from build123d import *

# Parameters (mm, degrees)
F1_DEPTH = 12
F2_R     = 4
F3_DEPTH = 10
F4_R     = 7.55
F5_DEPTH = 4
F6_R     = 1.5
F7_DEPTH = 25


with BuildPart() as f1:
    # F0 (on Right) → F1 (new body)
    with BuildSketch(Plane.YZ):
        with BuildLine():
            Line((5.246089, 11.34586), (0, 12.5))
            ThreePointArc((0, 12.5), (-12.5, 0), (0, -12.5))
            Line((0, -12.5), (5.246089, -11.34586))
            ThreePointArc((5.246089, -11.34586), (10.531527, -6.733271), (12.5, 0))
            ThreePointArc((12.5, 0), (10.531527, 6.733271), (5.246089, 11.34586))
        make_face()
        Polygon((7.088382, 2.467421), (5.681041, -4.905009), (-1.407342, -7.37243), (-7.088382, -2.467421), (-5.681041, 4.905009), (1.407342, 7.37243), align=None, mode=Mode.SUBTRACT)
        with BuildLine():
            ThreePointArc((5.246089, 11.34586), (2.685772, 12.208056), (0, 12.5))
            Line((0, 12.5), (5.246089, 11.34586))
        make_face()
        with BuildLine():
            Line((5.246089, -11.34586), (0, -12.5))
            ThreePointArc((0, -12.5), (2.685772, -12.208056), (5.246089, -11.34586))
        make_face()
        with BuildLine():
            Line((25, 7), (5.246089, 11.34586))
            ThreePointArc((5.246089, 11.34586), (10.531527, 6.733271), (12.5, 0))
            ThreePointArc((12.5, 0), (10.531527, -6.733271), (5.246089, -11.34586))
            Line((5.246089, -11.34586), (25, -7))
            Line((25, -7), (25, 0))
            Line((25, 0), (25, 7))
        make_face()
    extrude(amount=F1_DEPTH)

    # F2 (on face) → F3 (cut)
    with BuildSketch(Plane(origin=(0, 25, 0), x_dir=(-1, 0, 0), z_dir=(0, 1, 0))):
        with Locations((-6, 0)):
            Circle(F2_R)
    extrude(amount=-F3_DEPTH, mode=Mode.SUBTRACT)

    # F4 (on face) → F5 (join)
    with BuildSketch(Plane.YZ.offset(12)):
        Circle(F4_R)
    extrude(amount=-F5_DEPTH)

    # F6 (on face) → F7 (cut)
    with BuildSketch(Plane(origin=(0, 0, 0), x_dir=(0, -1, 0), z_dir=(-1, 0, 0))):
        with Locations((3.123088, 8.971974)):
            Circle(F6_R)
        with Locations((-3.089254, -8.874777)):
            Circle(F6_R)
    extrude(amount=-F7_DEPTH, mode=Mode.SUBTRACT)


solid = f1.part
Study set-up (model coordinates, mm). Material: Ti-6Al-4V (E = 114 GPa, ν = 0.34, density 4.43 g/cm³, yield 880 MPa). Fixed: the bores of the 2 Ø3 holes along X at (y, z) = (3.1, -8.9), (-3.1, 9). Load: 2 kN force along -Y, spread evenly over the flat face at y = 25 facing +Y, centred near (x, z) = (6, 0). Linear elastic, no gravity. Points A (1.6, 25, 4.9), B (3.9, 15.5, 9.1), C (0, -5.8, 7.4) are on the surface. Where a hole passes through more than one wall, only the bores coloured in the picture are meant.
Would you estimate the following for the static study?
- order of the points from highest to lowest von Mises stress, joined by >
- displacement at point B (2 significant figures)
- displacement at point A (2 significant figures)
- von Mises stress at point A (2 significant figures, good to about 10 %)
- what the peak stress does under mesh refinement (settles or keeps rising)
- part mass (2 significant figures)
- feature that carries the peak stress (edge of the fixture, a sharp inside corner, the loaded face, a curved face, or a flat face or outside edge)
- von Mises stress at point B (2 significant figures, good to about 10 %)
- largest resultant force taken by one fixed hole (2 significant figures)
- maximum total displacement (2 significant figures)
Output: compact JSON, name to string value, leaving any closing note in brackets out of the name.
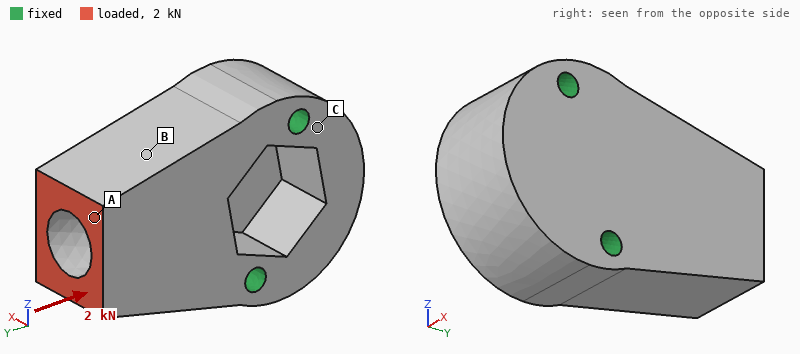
{"order of the points from highest to lowest von Mises stress, joined by >": "A > B > C", "displacement at point B": "2.2 µm", "displacement at point A": "3.7 µm", "von Mises stress at point A": "15 MPa", "what the peak stress does under mesh refinement": "keeps rising", "part mass": "31 g", "feature that carries the peak stress": "edge of the fixture", "von Mises stress at point B": "11 MPa", "largest resultant force taken by one fixed hole": "1.0 kN", "maximum total displacement": "4.0 µm"}
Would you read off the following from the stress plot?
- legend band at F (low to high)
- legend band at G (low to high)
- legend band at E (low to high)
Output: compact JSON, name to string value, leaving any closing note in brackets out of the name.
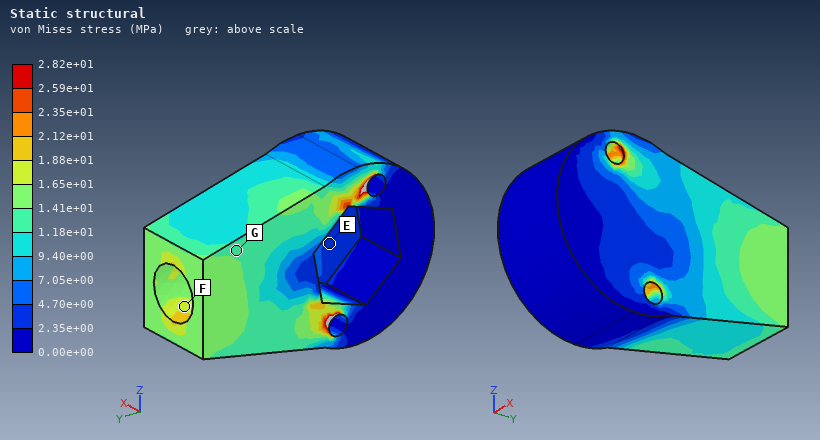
{"legend band at F": "1.65e+01 to 1.88e+01 MPa", "legend band at G": "1.18e+01 to 1.41e+01 MPa", "legend band at E": "2.35e+00 to 4.70e+00 MPa"}
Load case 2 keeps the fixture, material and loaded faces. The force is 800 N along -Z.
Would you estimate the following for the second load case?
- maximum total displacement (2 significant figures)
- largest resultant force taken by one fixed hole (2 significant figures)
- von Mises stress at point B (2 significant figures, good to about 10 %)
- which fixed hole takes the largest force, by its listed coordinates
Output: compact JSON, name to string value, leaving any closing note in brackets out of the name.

{"maximum total displacement": "7.6 µm", "largest resultant force taken by one fixed hole": "1.1 kN", "von Mises stress at point B": "17 MPa", "which fixed hole takes the largest force, by its listed coordinates": "(3.1, -8.9)"}
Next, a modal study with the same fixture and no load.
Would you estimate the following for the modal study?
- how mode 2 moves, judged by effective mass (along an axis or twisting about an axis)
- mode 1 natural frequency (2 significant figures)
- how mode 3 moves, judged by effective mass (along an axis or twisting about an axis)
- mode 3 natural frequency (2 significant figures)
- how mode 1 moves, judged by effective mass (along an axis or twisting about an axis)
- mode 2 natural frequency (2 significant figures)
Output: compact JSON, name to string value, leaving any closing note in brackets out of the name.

{"how mode 2 moves, judged by effective mass": "along Z", "mode 1 natural frequency": "15 kHz", "how mode 3 moves, judged by effective mass": "twisting about Y", "mode 3 natural frequency": "32 kHz", "how mode 1 moves, judged by effective mass": "along X", "mode 2 natural frequency": "25 kHz"}
